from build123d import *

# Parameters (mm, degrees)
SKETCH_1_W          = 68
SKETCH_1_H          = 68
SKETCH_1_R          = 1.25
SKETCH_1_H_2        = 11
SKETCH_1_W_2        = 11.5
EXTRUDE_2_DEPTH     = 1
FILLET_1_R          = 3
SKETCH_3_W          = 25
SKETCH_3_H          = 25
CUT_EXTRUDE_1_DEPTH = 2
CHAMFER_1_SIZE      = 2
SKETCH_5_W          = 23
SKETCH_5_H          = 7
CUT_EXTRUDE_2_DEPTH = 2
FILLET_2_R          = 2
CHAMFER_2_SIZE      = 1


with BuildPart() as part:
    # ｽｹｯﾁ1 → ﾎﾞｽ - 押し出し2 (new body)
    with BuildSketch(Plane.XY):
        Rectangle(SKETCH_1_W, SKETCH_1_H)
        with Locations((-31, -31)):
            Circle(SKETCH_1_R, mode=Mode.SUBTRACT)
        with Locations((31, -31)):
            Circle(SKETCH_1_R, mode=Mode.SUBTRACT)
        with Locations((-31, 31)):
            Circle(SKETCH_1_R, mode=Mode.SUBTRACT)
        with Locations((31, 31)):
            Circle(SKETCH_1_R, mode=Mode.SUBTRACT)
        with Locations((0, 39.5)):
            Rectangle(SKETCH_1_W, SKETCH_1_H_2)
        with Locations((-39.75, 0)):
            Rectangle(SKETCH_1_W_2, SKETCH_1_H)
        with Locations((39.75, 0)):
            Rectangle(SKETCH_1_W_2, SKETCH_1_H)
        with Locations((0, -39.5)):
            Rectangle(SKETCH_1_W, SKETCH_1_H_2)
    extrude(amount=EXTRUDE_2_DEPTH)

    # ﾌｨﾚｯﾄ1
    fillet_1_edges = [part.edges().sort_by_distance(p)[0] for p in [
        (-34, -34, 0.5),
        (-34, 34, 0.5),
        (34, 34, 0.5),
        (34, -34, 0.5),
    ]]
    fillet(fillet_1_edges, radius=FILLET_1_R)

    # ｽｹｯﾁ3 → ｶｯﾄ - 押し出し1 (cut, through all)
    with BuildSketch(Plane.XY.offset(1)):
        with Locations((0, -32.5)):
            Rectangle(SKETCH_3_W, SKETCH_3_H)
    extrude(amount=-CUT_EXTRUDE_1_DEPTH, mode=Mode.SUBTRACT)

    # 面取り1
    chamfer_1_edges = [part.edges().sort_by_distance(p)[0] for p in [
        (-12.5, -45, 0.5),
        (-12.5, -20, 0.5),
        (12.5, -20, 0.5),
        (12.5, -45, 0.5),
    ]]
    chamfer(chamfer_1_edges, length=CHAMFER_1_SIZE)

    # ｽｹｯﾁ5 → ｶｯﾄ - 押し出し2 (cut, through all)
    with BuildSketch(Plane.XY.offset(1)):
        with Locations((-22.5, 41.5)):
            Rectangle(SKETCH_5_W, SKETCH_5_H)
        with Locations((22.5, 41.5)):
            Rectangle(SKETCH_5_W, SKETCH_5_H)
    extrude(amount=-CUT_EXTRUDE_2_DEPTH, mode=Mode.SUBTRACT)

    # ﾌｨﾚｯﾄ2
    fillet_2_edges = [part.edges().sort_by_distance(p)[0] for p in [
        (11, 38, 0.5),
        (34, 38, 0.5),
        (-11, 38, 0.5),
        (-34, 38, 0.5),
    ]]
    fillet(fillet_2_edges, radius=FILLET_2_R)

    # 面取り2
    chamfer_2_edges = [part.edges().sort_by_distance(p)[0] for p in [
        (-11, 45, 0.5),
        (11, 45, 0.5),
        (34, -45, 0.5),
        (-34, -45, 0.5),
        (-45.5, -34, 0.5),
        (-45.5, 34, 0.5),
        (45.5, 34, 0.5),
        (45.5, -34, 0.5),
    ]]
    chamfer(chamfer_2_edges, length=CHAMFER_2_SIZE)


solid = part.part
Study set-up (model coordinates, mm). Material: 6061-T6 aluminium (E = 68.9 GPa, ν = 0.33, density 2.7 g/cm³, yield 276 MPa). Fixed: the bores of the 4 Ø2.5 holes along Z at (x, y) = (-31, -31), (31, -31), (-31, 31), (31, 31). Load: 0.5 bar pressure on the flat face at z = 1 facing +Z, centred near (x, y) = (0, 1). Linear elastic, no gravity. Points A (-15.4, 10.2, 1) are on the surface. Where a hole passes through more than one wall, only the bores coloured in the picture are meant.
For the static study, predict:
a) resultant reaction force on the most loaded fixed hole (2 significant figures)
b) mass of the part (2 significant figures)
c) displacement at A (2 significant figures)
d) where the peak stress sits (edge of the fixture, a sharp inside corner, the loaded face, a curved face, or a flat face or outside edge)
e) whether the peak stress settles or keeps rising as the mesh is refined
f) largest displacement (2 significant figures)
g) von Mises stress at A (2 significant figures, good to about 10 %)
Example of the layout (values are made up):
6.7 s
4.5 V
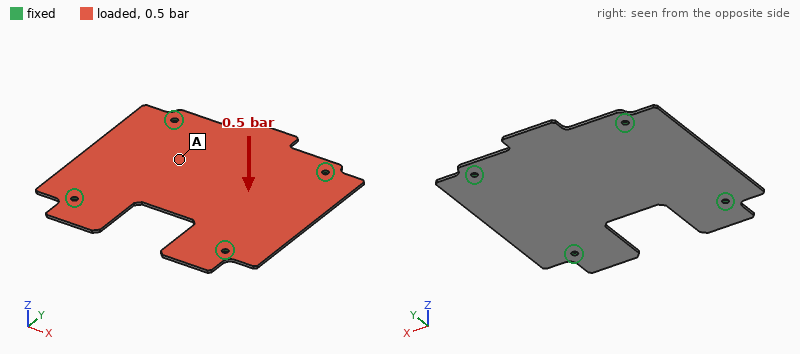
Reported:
87 N
18 g
0.62 mm
edge of the fixture
keeps rising
0.79 mm
42 MPa
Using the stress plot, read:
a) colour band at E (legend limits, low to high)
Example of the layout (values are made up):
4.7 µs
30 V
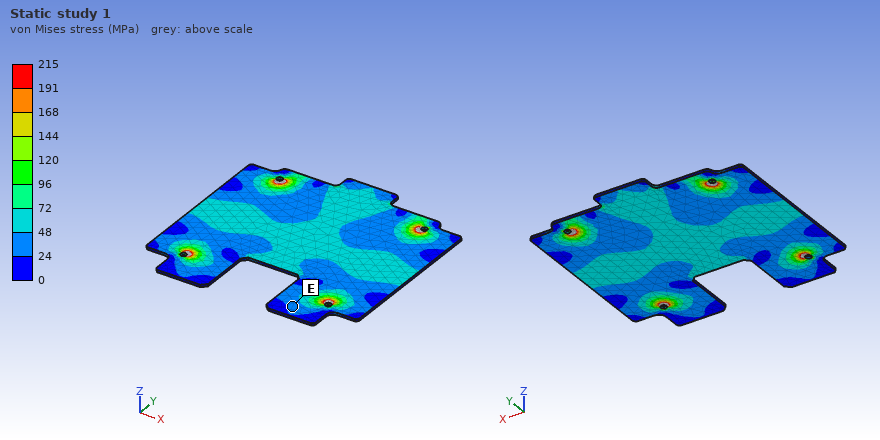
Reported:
24 to 48 MPa
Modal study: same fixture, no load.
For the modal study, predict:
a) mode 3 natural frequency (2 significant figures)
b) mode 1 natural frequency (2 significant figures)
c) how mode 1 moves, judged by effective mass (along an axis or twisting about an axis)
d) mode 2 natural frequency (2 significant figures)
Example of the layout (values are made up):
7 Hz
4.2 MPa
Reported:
1300 Hz
930 Hz
along Z
1300 Hz
